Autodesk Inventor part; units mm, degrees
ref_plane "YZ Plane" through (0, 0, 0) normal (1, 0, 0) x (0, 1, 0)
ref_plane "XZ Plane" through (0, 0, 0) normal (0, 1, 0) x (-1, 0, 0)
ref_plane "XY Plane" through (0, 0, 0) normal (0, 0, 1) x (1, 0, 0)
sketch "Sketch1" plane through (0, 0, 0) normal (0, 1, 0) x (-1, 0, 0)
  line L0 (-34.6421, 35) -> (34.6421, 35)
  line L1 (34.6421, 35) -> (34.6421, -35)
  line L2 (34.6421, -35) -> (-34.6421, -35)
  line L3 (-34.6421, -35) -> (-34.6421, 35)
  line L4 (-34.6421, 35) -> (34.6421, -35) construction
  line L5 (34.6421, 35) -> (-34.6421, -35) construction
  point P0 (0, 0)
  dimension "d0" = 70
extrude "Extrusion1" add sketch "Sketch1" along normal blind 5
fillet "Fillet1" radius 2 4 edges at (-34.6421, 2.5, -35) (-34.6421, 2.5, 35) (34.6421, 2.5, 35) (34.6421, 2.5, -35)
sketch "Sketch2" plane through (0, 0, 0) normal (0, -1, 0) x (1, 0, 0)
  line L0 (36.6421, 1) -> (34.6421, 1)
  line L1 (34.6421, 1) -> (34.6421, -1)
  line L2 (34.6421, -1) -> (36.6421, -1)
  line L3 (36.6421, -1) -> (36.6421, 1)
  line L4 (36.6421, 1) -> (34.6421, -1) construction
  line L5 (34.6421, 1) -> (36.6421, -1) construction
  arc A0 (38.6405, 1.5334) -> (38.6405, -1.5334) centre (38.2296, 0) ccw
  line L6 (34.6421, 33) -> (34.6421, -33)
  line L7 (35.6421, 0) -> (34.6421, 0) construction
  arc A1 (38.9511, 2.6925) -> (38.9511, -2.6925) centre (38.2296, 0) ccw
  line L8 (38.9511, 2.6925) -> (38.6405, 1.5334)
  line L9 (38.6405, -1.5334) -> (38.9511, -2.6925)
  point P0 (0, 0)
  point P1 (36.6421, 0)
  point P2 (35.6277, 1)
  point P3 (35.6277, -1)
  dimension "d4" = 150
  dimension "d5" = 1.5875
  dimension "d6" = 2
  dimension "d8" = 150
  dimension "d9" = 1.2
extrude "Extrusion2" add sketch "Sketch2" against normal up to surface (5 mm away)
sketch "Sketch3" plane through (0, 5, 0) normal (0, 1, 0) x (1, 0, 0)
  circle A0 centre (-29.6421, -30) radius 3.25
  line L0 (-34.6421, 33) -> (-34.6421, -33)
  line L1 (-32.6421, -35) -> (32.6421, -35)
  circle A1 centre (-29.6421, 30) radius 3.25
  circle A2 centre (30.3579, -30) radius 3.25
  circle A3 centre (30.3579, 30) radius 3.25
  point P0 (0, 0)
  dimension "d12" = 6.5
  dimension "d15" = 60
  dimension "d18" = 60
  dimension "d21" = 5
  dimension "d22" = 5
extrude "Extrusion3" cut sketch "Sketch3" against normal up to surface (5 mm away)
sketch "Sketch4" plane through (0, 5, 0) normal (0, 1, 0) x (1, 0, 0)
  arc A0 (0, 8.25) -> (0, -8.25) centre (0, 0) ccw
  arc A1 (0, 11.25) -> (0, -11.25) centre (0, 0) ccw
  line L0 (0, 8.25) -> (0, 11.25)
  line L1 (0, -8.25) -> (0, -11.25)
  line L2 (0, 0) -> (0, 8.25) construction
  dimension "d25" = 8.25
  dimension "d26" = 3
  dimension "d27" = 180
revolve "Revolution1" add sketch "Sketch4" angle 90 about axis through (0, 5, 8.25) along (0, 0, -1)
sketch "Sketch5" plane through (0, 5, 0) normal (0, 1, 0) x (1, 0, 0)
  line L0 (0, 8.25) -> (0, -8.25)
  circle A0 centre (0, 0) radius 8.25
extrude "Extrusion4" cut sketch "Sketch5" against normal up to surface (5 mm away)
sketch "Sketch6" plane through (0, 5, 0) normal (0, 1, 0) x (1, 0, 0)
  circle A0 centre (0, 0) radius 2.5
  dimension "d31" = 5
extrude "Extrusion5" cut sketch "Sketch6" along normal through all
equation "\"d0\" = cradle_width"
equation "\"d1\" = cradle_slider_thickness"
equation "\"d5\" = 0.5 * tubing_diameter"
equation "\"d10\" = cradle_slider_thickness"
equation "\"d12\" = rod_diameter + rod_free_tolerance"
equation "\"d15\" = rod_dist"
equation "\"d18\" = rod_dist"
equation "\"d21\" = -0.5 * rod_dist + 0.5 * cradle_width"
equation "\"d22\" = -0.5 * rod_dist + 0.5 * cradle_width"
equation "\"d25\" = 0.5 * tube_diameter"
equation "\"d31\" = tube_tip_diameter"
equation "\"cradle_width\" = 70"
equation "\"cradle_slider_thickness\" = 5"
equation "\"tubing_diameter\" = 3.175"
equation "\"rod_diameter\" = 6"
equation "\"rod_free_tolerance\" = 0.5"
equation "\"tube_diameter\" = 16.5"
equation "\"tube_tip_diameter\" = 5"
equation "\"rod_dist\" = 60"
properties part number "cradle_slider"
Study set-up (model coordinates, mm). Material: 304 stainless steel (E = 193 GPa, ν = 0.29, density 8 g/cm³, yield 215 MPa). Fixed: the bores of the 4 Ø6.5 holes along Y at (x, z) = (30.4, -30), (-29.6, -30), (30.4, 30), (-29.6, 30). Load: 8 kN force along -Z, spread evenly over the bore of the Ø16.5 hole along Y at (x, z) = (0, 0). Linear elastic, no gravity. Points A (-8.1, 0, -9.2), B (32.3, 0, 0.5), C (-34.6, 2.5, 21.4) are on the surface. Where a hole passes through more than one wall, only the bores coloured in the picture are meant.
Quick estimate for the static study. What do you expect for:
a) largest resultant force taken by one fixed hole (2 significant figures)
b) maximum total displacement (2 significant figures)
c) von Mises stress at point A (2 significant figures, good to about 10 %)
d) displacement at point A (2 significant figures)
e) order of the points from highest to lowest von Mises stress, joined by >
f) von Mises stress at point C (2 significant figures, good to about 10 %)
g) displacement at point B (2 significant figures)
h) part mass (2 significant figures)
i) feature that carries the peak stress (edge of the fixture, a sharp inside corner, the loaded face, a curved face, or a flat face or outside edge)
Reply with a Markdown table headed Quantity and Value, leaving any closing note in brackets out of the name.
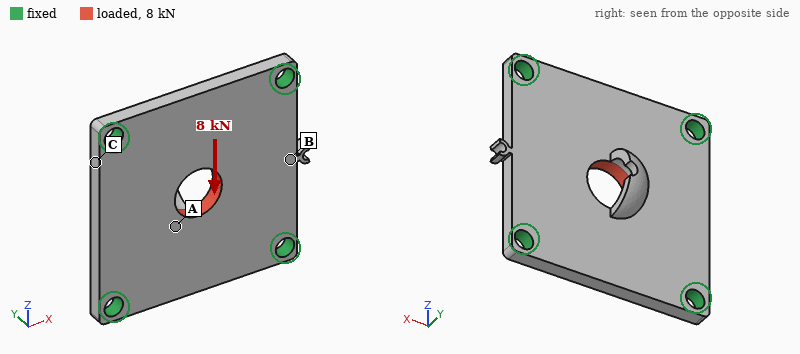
| Quantity | Value |
|---|---|
| largest resultant force taken by one fixed hole | 2.3 kN |
| maximum total displacement | 6.2 µm |
| von Mises stress at point A | 27 MPa |
| displacement at point A | 5.0 µm |
| order of the points from highest to lowest von Mises stress, joined by > | A > C > B |
| von Mises stress at point C | 15 MPa |
| displacement at point B | 1.7 µm |
| part mass | 190 g |
| feature that carries the peak stress | edge of the fixture |
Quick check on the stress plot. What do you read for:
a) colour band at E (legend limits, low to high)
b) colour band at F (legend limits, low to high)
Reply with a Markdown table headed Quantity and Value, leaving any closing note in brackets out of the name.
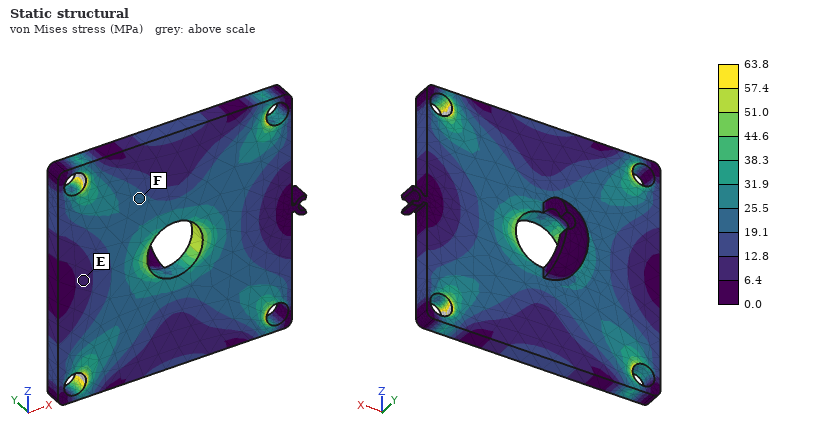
| Quantity | Value |
|---|---|
| colour band at E | 6.4 to 12.8 MPa |
| colour band at F | 19.1 to 25.5 MPa |
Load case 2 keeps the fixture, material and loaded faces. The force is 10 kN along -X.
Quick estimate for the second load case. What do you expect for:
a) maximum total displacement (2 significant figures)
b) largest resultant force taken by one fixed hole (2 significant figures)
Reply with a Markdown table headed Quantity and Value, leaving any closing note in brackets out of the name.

| Quantity | Value |
|---|---|
| maximum total displacement | 7.9 µm |
| largest resultant force taken by one fixed hole | 2.9 kN |
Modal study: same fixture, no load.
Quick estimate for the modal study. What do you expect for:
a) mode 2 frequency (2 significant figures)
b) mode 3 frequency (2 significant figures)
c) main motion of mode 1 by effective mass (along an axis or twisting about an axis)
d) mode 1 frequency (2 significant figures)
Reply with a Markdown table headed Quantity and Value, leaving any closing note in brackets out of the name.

| Quantity | Value |
|---|---|
| mode 2 frequency | 8000 Hz |
| mode 3 frequency | 8000 Hz |
| main motion of mode 1 by effective mass | along Y |
| mode 1 frequency | 4800 Hz |
